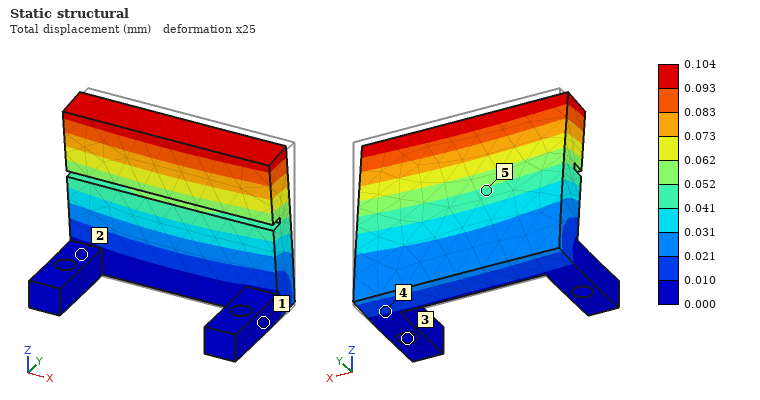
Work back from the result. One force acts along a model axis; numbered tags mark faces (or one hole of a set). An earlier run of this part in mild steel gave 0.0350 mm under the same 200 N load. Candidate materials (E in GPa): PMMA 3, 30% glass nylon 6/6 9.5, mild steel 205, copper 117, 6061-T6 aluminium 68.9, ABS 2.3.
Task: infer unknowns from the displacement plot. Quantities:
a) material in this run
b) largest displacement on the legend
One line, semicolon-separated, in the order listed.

6061-T6 aluminium; 0.104 mm
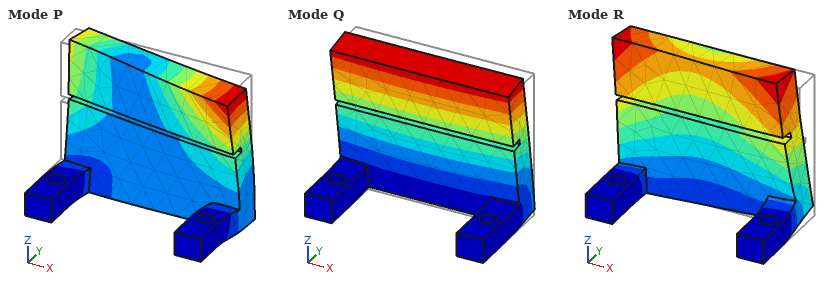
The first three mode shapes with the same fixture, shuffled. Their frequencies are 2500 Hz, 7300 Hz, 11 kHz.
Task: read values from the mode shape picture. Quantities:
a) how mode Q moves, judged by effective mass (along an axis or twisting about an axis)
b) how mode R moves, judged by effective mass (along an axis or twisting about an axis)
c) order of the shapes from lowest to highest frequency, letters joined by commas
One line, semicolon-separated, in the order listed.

along Y; along X; Q, R, P
